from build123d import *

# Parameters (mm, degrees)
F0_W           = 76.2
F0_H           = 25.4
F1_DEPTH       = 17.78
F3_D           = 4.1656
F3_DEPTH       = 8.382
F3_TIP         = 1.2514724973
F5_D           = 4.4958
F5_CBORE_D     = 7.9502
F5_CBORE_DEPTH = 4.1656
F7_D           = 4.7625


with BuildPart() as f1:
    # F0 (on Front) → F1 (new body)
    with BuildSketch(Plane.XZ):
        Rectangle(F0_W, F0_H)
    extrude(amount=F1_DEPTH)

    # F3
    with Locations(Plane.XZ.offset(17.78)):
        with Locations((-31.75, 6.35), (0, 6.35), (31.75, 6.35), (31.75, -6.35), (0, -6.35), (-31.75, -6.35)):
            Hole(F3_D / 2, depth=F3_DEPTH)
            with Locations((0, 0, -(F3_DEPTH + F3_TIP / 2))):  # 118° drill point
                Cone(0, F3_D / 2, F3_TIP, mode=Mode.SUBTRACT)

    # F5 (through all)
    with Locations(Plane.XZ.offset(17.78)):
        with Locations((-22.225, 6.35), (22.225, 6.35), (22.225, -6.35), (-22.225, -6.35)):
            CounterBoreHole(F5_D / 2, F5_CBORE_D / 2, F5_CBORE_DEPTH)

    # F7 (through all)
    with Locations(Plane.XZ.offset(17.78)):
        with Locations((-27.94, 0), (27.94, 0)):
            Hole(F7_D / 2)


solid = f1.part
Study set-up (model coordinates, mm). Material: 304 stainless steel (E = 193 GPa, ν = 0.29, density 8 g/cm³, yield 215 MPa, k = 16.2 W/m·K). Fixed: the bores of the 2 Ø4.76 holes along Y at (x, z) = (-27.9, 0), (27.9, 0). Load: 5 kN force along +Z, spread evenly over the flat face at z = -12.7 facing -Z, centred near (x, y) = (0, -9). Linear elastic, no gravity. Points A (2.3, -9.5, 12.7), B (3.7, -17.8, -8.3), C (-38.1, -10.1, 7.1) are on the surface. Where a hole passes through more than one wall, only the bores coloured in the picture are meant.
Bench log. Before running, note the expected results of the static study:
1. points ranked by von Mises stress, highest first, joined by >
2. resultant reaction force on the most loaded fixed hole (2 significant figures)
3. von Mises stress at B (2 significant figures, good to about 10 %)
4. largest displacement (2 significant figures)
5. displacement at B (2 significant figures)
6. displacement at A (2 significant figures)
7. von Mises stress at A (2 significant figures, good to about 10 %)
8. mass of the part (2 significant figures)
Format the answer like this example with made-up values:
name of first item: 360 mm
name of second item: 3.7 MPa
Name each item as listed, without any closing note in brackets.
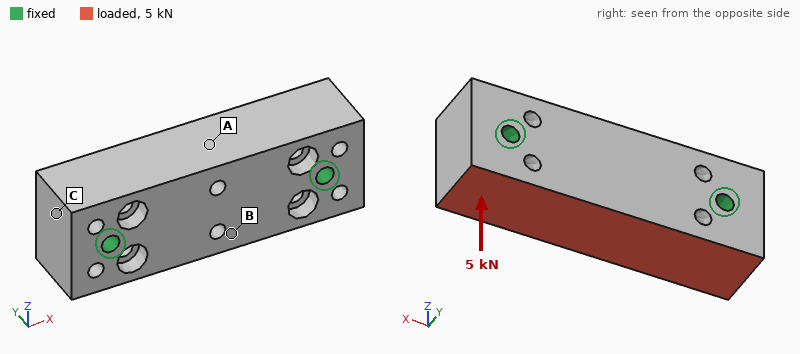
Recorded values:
points ranked by von Mises stress, highest first, joined by >: A > B > C
resultant reaction force on the most loaded fixed hole: 2.5 kN
von Mises stress at B: 5.9 MPa
largest displacement: 2.6 µm
displacement at B: 2.5 µm
displacement at A: 2.1 µm
von Mises stress at A: 9.4 MPa
mass of the part: 250 g
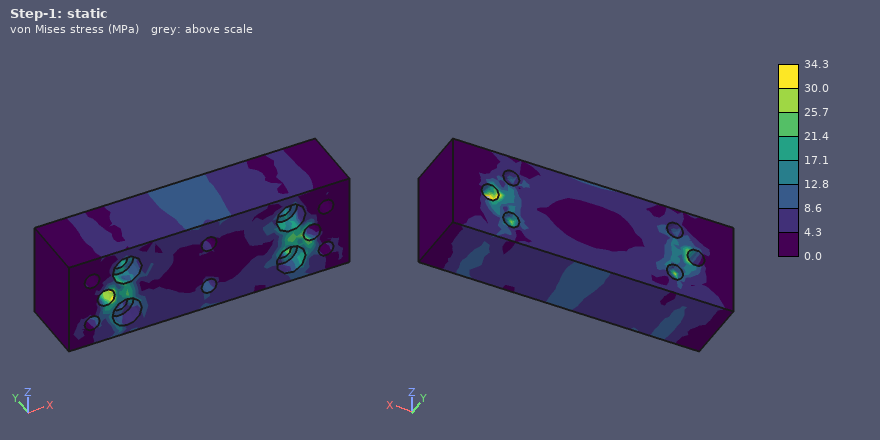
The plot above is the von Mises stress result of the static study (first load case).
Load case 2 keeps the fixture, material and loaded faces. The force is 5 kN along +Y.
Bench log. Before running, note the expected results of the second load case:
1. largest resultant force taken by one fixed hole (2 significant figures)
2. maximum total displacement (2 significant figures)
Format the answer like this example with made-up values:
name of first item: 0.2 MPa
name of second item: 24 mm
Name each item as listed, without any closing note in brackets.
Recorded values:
largest resultant force taken by one fixed hole: 2.5 kN
maximum total displacement: 7.6 µm
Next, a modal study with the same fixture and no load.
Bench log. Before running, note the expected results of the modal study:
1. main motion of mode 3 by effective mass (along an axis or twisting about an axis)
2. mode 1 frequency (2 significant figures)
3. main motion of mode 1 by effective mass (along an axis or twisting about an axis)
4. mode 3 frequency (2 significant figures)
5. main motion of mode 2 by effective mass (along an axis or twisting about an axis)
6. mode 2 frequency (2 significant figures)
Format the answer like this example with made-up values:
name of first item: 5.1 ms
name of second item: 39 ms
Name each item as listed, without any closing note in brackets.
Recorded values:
main motion of mode 3 by effective mass: twisting about X
mode 1 frequency: 15 kHz
main motion of mode 1 by effective mass: along Z
mode 3 frequency: 18 kHz
main motion of mode 2 by effective mass: along Y
mode 2 frequency: 16 kHz
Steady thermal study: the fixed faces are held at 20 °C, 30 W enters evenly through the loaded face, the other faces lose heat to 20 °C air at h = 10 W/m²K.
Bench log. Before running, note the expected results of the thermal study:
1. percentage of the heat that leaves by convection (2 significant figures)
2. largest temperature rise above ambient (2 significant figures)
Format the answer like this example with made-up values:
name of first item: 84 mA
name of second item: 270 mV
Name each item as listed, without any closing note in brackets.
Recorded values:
percentage of the heat that leaves by convection: 4.4 %
largest temperature rise above ambient: 43 K
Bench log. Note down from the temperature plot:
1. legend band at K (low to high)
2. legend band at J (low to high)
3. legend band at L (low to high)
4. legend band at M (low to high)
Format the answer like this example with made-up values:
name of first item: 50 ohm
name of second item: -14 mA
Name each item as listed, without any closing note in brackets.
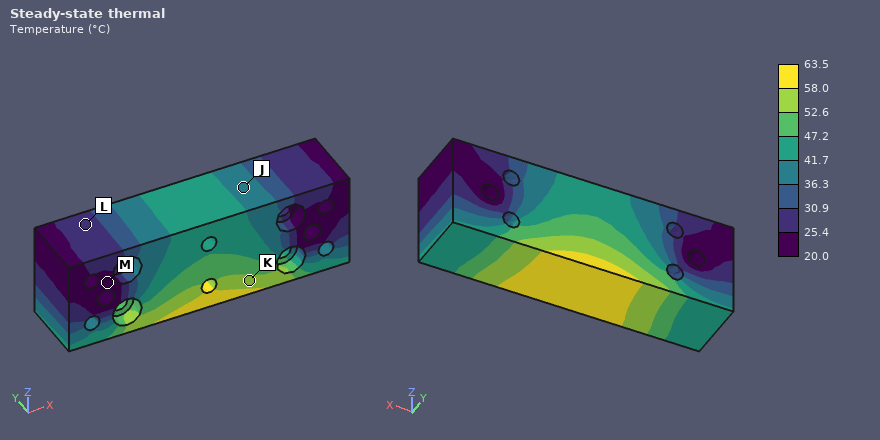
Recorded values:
legend band at K: 52.6 to 58.0 °C
legend band at J: 36.3 to 41.7 °C
legend band at L: 25.4 to 30.9 °C
legend band at M: 20.0 to 25.4 °C
